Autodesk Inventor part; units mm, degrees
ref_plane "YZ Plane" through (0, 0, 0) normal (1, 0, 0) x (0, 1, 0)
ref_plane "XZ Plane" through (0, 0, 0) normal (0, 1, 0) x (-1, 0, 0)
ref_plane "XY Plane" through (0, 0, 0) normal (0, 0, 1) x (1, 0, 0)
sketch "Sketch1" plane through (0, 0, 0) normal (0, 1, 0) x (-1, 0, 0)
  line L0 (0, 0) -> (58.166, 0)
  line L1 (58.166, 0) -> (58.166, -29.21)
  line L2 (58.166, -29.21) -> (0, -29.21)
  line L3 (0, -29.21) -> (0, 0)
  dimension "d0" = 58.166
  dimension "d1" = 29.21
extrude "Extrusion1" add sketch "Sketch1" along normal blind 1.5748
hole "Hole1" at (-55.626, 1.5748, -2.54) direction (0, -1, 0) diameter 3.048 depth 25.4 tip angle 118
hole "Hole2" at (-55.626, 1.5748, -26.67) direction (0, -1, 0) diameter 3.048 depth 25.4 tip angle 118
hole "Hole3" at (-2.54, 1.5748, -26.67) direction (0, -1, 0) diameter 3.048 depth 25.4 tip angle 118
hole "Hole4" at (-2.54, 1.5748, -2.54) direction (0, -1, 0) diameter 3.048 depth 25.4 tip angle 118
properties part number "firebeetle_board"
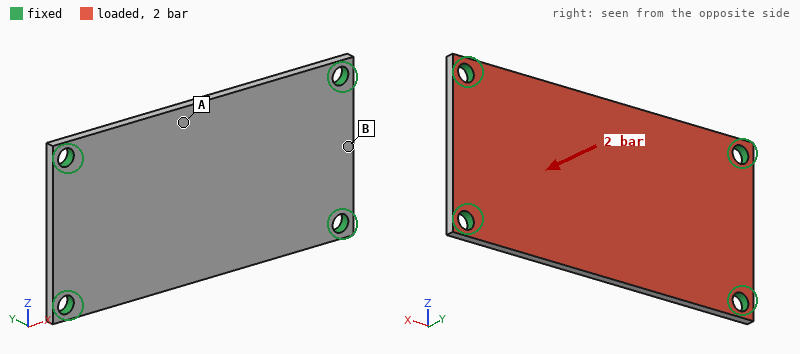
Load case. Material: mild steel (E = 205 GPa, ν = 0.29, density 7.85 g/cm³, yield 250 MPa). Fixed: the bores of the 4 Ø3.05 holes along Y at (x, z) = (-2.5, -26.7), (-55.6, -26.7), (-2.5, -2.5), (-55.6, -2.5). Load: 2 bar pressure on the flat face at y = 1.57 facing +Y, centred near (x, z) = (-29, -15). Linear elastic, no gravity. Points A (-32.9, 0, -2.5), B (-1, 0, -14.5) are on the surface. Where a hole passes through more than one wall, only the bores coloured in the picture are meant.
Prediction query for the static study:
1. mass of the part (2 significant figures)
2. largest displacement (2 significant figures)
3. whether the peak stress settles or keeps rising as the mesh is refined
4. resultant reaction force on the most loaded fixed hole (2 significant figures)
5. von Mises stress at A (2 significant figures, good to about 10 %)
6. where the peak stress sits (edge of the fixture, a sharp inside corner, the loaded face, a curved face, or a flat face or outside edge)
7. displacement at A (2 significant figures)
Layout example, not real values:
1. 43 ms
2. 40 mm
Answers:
1. 21 g
2. 70 µm
3. keeps rising
4. 84 N
5. 58 MPa
6. edge of the fixture
7. 66 µm
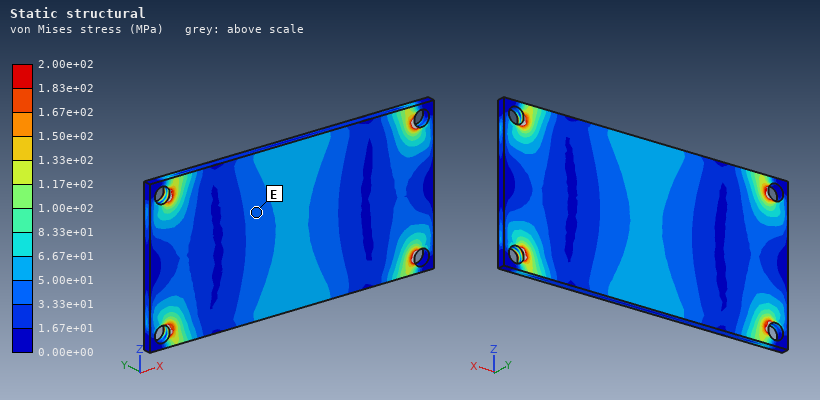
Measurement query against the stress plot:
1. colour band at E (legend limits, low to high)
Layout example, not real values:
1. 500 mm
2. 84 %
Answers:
1. 3.33e+01 to 5.00e+01 MPa
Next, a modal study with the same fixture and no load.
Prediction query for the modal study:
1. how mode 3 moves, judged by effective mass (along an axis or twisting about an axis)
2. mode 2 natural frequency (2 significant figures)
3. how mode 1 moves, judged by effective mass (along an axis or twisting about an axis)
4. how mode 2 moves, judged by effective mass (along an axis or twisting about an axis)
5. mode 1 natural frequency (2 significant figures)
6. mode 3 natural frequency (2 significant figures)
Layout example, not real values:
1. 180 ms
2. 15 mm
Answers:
1. twisting about Z
2. 4800 Hz
3. along Y
4. twisting about X
5. 2800 Hz
6. 7600 Hz
